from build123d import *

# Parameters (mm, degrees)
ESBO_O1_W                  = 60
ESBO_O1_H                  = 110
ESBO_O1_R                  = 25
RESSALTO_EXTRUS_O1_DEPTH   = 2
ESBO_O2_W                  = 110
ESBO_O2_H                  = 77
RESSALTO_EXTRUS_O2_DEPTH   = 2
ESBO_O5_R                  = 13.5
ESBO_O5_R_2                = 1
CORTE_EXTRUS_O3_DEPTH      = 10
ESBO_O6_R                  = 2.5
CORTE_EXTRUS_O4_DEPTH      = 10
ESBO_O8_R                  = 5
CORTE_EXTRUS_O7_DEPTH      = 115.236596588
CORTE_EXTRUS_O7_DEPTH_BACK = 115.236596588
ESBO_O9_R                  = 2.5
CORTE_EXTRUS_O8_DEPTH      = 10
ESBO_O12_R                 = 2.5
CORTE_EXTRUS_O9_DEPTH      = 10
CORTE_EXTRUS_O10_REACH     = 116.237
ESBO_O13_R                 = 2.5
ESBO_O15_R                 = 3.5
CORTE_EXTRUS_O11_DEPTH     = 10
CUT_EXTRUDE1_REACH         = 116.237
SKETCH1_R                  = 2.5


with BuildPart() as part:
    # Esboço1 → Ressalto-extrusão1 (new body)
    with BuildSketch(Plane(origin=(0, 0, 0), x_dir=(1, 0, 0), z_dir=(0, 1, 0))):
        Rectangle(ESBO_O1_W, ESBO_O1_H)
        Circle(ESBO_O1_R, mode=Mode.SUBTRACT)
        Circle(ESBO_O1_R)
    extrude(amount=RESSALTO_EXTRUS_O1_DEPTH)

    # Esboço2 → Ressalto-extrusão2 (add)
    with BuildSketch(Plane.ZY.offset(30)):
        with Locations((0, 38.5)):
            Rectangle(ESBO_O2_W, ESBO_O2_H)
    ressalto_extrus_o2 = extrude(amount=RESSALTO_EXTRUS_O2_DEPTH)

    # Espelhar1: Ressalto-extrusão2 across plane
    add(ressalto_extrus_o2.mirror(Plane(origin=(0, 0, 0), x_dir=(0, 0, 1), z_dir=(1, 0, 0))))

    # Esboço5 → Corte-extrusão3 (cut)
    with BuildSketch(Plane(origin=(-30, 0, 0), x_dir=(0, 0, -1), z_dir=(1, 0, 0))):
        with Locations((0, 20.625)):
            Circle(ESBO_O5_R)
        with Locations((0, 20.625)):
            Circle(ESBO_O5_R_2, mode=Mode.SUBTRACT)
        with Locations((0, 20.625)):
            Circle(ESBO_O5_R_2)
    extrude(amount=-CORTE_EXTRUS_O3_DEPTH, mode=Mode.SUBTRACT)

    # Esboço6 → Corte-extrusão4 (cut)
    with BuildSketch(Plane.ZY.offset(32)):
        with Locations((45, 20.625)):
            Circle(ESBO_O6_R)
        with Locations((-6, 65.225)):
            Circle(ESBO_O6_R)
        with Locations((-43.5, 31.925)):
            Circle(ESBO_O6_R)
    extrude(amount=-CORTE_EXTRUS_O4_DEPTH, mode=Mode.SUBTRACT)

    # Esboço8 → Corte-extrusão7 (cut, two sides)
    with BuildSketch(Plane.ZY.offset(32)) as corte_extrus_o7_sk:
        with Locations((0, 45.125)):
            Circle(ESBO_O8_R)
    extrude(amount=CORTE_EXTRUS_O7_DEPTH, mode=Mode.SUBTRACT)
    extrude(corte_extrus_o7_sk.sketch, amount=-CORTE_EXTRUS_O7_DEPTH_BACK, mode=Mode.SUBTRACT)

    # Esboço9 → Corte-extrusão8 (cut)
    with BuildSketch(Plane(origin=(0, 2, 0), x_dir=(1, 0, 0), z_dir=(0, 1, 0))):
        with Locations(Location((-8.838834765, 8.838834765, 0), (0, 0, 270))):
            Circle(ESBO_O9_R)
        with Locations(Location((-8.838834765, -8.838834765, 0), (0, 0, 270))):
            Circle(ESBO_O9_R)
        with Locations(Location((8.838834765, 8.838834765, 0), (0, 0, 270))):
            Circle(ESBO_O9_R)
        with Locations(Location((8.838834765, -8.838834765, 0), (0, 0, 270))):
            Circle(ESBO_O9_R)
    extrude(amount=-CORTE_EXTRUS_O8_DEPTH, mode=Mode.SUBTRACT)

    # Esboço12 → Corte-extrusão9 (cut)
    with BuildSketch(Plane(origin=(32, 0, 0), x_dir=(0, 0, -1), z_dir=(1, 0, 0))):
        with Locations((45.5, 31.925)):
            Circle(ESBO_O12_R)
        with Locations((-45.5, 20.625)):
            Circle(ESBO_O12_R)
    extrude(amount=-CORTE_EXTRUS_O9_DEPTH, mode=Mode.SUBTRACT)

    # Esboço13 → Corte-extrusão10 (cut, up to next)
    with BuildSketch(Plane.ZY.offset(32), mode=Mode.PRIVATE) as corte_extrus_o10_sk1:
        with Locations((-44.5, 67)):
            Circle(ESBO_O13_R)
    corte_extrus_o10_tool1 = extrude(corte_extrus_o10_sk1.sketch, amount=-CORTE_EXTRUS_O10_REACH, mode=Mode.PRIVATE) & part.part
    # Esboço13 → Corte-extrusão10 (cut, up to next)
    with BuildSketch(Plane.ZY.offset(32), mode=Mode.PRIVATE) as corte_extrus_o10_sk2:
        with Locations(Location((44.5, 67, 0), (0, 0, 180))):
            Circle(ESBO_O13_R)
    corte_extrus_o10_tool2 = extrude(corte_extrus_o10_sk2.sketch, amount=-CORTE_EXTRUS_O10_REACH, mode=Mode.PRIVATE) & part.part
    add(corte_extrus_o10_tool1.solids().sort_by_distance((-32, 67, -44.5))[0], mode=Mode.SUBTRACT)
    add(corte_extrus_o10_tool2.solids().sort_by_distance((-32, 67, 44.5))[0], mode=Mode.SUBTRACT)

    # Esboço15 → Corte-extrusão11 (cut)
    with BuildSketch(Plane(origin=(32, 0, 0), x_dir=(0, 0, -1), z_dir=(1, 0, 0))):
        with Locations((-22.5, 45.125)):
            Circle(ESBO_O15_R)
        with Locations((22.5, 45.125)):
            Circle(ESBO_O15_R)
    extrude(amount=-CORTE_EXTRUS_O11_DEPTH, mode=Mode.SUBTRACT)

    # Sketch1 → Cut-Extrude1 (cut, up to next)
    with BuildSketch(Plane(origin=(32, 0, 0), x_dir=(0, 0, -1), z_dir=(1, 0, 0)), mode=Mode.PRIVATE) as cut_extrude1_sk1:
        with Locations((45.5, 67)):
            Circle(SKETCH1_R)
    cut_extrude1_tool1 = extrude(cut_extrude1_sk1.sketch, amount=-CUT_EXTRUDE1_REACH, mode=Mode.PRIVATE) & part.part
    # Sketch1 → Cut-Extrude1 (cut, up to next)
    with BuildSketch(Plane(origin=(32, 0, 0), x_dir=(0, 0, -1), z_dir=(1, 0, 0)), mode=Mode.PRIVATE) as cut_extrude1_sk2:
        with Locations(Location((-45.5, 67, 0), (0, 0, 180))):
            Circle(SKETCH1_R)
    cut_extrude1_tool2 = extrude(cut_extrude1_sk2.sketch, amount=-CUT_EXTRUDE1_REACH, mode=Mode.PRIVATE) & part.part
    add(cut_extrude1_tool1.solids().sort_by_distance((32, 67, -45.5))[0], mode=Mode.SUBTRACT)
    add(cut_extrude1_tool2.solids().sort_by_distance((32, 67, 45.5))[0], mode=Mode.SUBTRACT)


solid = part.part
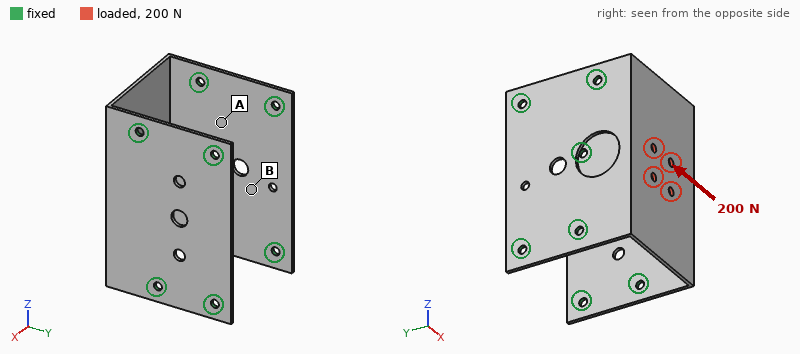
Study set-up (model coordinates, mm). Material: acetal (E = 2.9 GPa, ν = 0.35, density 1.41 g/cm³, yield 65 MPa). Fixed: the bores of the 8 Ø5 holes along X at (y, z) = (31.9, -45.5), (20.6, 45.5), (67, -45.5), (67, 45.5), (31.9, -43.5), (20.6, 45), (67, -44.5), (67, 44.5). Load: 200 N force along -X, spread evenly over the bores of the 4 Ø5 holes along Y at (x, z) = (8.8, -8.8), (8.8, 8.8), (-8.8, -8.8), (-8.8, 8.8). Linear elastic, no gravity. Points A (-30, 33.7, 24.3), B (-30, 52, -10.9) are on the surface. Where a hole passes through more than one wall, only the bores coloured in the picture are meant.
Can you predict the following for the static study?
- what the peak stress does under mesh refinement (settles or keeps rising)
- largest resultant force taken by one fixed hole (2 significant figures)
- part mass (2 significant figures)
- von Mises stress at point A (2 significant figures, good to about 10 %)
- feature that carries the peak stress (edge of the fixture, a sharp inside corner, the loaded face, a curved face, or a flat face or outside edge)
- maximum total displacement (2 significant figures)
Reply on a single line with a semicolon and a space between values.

keeps rising; 100 N; 63 g; 4.6 MPa; edge of the fixture; 1.4 mm
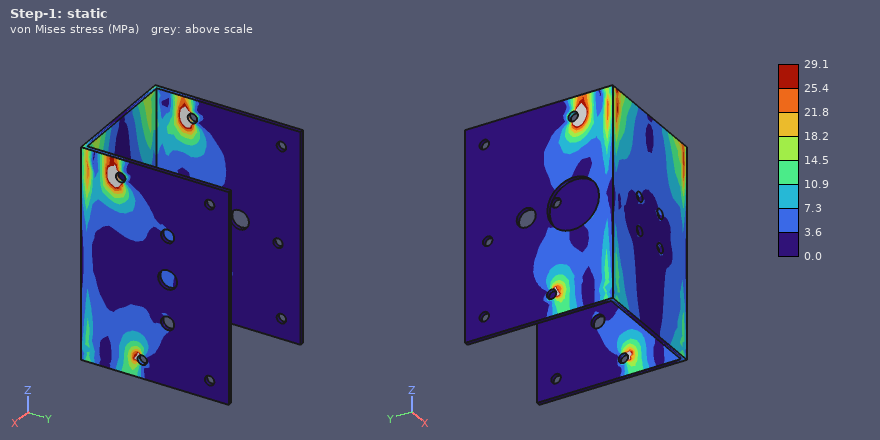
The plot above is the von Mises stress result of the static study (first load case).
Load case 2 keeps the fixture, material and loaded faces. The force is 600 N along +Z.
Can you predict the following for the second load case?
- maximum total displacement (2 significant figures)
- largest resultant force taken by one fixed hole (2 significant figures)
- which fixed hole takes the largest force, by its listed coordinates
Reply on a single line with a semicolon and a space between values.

0.12 mm; 190 N; (20.6, 45)
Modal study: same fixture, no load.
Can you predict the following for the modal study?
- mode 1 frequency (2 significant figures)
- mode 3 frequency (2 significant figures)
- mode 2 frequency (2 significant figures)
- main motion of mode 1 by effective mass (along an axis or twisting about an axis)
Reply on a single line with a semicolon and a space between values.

370 Hz; 410 Hz; 400 Hz; along X
